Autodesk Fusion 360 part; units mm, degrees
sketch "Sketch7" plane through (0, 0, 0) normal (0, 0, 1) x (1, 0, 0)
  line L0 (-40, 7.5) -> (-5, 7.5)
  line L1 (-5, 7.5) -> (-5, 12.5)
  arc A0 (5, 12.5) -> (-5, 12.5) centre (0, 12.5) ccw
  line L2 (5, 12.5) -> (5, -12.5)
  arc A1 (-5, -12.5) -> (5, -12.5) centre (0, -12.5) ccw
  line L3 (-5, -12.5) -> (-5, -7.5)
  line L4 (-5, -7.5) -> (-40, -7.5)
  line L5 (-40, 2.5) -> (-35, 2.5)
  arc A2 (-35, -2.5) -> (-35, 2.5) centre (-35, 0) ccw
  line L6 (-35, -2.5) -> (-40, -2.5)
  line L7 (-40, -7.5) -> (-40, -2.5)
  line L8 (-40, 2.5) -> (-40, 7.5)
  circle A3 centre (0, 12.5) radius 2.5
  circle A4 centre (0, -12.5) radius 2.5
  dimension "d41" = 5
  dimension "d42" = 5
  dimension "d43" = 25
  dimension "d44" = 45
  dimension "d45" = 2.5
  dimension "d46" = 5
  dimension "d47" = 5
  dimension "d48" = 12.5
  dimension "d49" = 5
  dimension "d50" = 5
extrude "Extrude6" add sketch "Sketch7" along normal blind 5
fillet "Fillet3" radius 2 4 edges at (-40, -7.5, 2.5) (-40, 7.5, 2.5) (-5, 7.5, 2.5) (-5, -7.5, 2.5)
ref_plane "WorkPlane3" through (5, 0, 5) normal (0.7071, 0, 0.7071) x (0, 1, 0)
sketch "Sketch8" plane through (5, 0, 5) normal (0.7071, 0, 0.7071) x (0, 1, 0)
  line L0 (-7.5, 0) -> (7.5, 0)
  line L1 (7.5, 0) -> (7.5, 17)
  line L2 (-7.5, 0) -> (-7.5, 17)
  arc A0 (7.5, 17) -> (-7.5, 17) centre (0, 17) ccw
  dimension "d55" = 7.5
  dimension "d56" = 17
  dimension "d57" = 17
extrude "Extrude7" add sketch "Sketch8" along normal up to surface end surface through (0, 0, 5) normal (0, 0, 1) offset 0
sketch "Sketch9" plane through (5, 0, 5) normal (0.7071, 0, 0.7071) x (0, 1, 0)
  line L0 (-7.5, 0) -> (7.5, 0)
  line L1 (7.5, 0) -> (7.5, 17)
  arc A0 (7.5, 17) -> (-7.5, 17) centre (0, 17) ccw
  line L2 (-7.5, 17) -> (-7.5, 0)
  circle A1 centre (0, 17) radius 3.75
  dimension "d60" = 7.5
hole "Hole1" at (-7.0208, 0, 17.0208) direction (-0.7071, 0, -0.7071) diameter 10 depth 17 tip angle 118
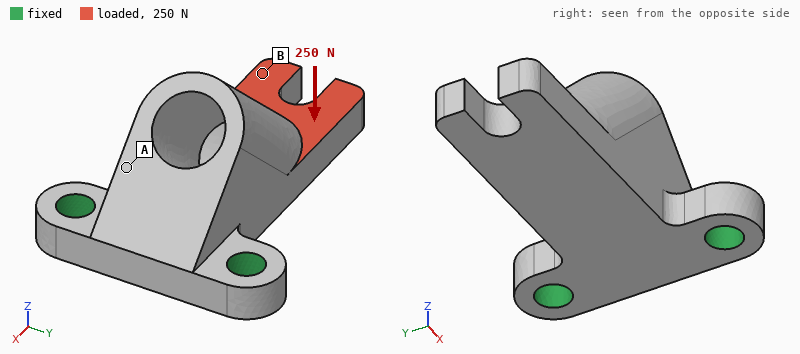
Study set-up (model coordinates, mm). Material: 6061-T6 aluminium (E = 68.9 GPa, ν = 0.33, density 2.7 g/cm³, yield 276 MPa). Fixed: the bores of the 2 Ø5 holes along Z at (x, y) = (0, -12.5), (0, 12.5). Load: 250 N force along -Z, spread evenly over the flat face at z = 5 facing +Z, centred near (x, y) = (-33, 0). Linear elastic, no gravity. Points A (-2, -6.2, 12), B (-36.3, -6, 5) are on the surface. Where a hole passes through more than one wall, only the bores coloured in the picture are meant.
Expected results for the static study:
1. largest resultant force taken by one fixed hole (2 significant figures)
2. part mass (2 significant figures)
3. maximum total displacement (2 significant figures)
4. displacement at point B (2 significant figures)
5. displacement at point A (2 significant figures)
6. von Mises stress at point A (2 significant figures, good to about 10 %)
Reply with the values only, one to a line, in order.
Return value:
160 N
17 g
0.13 mm
0.11 mm
0.024 mm
20 MPa
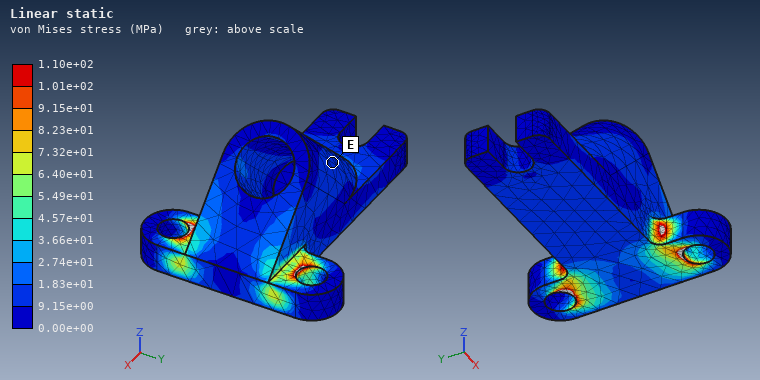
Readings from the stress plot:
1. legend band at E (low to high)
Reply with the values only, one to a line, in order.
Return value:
9.15e+00 to 1.83e+01 MPa
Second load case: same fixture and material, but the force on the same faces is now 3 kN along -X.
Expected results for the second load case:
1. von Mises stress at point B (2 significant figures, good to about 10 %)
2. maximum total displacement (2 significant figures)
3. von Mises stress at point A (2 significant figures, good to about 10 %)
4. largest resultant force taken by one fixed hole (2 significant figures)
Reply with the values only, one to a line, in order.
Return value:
64 MPa
0.14 mm
15 MPa
1.6 kN
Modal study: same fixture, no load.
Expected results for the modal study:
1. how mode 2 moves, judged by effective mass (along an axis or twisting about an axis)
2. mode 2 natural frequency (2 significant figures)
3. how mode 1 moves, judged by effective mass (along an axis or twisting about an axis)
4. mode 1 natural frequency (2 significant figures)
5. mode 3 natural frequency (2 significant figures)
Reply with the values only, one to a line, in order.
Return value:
along Y
8900 Hz
along Z
3800 Hz
16 kHz
